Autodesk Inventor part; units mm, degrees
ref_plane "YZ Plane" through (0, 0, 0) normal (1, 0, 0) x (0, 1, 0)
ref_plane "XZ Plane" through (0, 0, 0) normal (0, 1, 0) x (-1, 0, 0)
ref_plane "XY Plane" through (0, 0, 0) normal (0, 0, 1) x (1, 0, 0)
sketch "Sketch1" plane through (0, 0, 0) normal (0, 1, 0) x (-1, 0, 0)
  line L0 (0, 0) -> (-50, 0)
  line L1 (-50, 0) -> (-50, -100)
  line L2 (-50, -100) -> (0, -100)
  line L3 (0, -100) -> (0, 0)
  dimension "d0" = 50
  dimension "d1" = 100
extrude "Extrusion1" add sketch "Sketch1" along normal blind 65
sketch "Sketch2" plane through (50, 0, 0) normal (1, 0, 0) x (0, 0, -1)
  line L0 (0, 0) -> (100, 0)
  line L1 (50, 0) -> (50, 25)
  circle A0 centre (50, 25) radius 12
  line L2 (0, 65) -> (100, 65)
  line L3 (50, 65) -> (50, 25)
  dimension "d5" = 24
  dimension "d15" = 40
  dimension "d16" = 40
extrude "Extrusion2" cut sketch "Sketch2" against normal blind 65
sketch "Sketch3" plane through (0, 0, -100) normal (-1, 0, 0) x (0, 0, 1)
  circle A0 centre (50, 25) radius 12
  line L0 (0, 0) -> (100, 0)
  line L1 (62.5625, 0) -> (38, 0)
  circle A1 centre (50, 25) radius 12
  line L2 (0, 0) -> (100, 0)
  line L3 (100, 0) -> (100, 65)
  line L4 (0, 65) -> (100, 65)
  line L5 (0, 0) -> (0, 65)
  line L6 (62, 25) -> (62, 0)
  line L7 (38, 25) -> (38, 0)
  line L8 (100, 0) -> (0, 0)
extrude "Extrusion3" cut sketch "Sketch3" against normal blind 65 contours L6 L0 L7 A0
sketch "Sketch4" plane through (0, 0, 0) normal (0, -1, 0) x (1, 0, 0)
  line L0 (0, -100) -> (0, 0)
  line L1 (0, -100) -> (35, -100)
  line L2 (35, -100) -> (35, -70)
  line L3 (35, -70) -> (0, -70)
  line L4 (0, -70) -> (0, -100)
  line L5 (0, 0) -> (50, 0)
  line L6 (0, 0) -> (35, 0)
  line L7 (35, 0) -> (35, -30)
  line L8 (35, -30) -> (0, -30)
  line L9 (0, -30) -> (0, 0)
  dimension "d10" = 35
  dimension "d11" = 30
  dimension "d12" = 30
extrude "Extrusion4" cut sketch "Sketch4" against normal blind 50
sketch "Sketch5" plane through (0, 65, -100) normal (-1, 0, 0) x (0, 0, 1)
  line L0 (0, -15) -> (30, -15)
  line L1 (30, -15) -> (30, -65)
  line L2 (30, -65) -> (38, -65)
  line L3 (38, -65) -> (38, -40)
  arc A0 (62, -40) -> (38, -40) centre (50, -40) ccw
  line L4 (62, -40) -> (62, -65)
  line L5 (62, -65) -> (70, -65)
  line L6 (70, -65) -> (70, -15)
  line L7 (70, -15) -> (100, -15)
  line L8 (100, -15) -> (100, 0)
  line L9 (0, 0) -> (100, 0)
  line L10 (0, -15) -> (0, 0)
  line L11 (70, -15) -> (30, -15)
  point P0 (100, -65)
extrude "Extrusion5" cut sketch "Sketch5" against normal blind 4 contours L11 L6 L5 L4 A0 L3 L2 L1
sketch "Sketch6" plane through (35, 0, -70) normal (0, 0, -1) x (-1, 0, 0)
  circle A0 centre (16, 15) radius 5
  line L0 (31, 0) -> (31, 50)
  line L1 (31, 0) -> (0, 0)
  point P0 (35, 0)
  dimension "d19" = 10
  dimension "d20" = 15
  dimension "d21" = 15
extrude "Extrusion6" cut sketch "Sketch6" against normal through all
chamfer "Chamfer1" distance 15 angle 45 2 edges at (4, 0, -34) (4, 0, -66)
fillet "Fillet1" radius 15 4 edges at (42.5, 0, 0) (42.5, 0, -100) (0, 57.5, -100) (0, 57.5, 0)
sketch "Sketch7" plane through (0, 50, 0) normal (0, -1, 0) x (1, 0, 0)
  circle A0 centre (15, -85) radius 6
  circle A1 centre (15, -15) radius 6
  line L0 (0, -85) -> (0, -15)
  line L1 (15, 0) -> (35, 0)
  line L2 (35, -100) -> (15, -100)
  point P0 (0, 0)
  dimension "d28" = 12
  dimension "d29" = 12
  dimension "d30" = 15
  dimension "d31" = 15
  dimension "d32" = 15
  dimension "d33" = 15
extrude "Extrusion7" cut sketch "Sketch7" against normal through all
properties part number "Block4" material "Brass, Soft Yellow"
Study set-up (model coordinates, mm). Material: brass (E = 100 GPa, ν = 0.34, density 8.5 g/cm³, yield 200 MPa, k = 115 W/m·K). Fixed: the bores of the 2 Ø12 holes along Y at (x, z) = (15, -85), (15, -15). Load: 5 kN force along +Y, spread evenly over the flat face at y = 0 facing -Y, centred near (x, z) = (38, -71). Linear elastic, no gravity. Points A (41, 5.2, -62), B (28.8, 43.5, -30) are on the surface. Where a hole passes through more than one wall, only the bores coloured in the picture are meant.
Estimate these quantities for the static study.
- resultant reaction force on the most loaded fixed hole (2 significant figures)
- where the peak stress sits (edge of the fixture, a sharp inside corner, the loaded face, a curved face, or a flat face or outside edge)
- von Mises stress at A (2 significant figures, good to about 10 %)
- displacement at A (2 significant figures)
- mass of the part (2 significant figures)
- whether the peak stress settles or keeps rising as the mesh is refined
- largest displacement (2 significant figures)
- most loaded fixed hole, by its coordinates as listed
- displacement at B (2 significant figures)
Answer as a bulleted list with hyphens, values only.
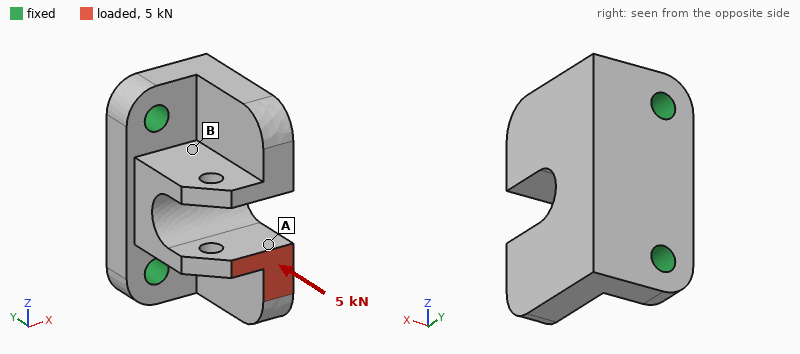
- 4.1 kN
- edge of the fixture
- 11 MPa
- 33 µm
- 1.4 kg
- keeps rising
- 40 µm
- (15, -85)
- 8.1 µm
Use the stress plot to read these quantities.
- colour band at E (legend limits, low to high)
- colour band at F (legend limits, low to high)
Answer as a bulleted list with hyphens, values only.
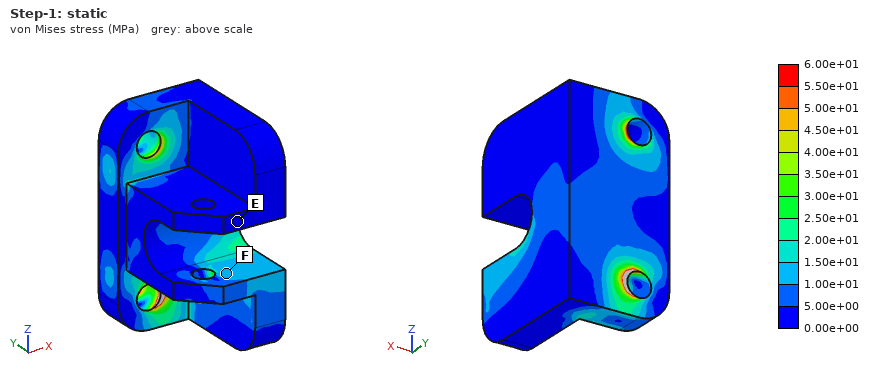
- 0.00e+00 to 5.00e+00 MPa
- 1.00e+01 to 1.50e+01 MPa
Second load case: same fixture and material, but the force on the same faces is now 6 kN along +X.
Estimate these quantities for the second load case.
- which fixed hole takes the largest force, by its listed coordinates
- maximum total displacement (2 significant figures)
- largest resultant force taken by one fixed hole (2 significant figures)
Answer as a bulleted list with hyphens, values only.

- (15, -85)
- 0.18 mm
- 4.8 kN
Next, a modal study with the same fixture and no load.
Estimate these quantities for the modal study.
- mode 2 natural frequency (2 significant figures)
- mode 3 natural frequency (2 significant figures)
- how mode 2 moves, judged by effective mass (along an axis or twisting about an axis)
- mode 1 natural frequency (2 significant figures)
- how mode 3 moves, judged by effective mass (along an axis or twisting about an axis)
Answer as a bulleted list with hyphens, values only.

- 3700 Hz
- 4400 Hz
- along Z
- 1900 Hz
- along Z
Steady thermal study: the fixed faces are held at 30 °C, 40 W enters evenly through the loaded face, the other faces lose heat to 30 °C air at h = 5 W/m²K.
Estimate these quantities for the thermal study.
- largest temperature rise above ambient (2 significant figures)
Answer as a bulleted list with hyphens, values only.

- 31 K
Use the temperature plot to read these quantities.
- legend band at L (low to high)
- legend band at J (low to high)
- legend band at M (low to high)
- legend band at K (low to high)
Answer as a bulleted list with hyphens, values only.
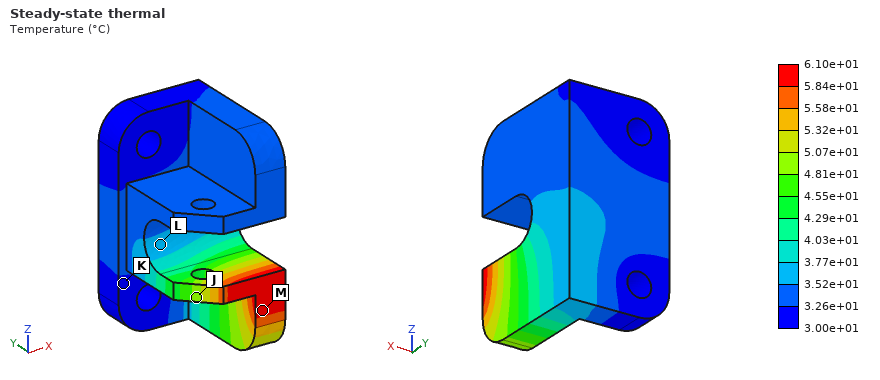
- 3.52e+01 to 3.77e+01 °C
- 4.81e+01 to 5.07e+01 °C
- 5.84e+01 to 6.10e+01 °C
- 3.00e+01 to 3.26e+01 °C
